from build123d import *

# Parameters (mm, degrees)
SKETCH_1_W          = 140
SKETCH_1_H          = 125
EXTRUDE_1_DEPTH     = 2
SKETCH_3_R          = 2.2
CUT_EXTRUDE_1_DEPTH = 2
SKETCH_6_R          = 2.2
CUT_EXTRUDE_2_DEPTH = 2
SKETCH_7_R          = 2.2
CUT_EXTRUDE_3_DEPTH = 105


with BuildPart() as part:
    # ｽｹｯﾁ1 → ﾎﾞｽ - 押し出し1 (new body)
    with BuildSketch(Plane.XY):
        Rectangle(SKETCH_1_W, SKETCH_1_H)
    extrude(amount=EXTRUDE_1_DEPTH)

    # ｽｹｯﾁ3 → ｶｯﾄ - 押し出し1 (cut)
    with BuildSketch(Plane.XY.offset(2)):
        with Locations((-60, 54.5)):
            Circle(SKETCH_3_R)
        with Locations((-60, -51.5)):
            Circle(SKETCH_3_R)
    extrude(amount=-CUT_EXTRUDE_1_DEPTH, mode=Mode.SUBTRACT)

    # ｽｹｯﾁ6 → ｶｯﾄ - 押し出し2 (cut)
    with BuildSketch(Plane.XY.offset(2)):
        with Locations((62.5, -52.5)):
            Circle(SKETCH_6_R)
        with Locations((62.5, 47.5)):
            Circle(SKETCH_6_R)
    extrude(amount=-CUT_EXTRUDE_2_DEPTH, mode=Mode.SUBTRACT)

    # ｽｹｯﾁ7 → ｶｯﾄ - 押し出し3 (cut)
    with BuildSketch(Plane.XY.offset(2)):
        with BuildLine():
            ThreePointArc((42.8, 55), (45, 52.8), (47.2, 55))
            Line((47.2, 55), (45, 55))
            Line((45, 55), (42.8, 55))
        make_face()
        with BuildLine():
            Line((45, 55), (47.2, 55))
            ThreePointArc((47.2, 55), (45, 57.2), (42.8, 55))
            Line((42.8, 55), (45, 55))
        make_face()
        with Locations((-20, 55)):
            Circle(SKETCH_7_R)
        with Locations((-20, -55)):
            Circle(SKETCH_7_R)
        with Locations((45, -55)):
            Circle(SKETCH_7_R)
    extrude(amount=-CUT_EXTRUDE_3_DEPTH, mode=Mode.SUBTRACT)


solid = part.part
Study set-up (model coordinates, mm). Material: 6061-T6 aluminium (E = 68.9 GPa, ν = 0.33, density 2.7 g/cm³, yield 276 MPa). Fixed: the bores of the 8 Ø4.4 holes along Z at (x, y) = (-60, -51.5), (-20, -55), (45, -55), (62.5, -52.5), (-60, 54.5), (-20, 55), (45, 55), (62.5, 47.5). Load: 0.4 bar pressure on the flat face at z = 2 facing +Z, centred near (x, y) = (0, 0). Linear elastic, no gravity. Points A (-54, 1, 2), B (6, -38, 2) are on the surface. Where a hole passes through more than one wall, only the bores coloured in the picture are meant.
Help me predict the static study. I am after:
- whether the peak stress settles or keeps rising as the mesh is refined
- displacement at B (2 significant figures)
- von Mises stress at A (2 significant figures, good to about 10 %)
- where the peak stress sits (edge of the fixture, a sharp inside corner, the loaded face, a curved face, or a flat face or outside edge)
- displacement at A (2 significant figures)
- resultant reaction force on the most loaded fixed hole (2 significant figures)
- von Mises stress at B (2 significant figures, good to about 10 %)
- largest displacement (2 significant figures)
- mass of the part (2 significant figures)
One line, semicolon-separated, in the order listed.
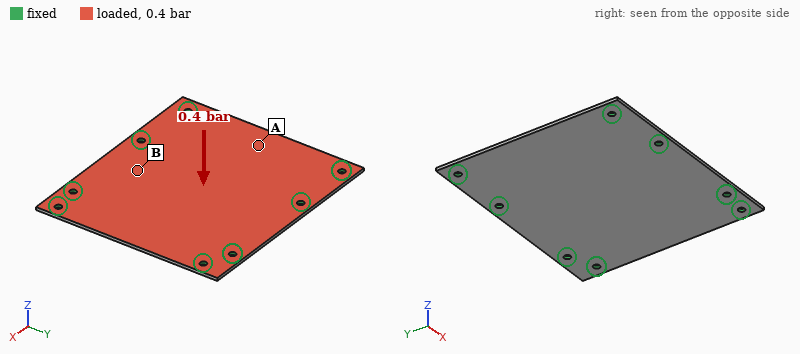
keeps rising; 0.18 mm; 29 MPa; edge of the fixture; 0.32 mm; 130 N; 15 MPa; 0.39 mm; 94 g
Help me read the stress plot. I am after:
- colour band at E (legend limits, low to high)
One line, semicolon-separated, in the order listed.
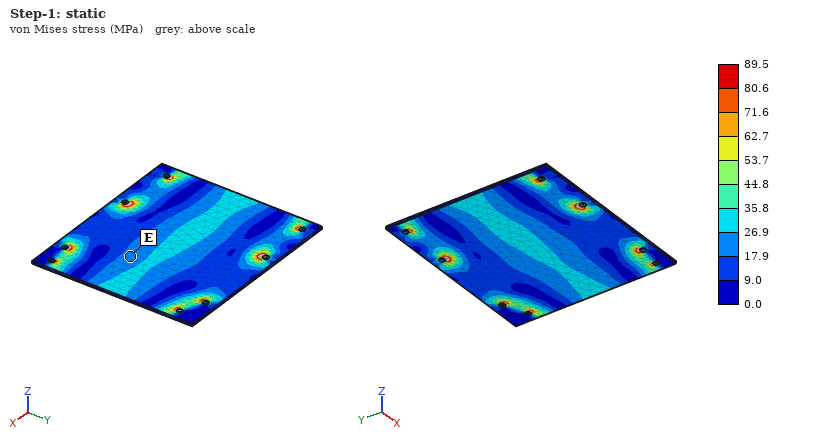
17.9 to 26.9 MPa
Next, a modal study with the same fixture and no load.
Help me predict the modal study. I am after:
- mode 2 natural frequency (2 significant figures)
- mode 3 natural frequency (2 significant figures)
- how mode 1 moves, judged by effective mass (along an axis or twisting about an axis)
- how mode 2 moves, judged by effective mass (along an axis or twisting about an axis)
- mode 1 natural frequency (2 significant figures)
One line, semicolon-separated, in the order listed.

1100 Hz; 1400 Hz; along Z; twisting about Y; 830 Hz
